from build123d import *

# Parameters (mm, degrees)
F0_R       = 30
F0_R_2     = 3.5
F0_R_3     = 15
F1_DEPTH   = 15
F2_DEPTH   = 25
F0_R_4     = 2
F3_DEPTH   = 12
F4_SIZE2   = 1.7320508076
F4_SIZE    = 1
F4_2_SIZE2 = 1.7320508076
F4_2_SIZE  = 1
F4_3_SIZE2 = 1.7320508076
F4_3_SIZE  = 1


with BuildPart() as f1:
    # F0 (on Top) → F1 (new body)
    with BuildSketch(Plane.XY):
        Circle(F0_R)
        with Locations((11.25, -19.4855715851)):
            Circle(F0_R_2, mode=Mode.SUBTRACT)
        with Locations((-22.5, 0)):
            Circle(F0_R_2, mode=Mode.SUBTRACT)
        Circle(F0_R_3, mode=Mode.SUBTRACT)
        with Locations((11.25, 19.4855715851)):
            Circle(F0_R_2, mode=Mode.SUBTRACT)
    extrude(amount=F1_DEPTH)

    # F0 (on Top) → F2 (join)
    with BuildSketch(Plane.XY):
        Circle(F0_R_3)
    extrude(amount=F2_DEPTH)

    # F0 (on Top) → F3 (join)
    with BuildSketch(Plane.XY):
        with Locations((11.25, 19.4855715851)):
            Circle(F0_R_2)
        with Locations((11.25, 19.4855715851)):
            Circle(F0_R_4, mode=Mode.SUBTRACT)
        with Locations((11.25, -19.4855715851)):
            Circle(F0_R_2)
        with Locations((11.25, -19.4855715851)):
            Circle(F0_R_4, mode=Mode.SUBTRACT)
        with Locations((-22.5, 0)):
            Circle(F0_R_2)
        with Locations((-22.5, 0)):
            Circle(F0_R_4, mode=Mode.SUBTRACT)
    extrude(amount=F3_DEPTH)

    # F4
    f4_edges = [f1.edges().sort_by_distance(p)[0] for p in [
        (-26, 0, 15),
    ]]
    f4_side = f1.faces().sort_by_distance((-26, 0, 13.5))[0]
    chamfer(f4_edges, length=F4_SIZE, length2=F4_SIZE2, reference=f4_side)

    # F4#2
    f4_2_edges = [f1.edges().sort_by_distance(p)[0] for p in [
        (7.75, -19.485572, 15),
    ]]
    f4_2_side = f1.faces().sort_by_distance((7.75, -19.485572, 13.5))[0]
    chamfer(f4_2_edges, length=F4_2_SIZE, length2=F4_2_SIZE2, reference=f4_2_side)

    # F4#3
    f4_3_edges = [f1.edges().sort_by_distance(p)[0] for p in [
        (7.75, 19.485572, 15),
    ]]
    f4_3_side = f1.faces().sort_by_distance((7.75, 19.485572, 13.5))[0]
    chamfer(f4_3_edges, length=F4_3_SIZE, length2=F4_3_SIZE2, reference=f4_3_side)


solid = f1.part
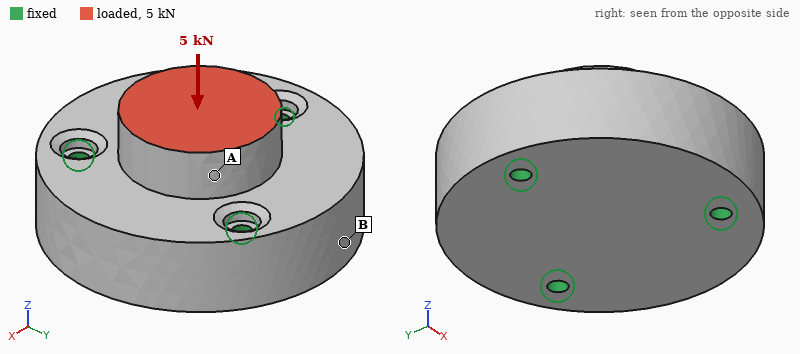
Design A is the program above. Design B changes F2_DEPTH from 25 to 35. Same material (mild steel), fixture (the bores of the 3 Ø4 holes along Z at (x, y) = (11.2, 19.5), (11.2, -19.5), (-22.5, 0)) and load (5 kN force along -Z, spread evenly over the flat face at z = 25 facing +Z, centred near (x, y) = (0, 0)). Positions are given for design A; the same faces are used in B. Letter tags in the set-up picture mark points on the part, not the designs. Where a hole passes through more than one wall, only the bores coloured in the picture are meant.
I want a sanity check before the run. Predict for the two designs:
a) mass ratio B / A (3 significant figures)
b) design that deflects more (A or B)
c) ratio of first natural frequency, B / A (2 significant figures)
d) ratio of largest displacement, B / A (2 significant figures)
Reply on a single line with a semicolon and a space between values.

1.15; B; 0.80; 1.2
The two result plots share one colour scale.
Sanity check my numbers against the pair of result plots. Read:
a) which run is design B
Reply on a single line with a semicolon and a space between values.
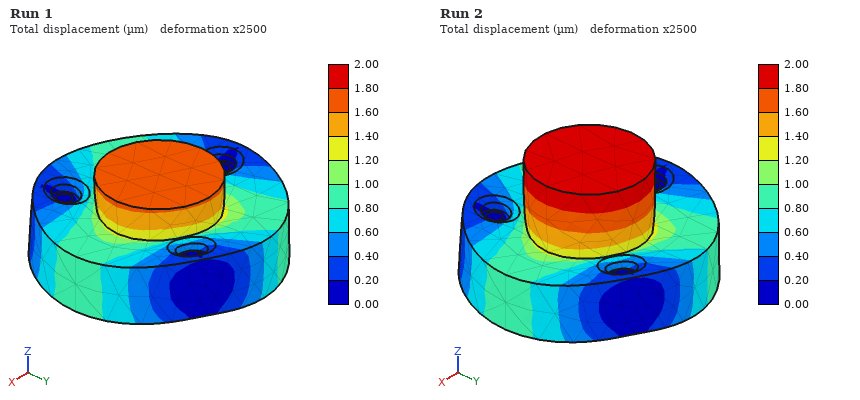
Run 2
